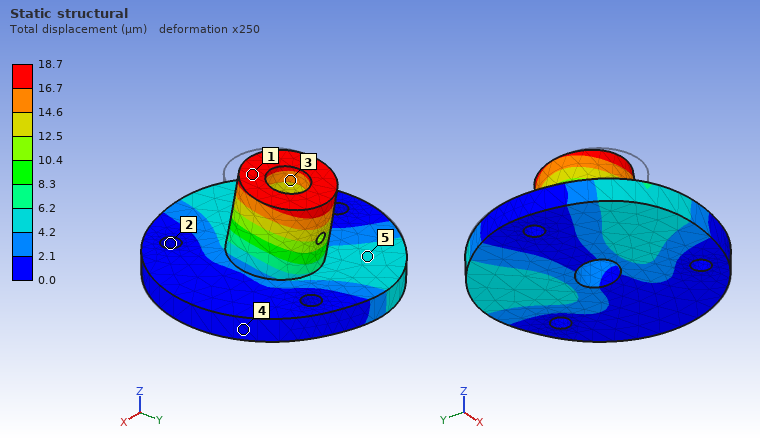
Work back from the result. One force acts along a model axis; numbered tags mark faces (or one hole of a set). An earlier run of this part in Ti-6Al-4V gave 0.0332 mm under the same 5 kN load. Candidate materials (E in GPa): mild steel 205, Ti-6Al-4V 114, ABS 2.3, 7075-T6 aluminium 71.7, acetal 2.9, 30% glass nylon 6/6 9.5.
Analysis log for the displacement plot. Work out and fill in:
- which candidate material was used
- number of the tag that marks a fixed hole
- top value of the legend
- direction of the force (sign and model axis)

mild steel
2
18.7 µm
+Y
